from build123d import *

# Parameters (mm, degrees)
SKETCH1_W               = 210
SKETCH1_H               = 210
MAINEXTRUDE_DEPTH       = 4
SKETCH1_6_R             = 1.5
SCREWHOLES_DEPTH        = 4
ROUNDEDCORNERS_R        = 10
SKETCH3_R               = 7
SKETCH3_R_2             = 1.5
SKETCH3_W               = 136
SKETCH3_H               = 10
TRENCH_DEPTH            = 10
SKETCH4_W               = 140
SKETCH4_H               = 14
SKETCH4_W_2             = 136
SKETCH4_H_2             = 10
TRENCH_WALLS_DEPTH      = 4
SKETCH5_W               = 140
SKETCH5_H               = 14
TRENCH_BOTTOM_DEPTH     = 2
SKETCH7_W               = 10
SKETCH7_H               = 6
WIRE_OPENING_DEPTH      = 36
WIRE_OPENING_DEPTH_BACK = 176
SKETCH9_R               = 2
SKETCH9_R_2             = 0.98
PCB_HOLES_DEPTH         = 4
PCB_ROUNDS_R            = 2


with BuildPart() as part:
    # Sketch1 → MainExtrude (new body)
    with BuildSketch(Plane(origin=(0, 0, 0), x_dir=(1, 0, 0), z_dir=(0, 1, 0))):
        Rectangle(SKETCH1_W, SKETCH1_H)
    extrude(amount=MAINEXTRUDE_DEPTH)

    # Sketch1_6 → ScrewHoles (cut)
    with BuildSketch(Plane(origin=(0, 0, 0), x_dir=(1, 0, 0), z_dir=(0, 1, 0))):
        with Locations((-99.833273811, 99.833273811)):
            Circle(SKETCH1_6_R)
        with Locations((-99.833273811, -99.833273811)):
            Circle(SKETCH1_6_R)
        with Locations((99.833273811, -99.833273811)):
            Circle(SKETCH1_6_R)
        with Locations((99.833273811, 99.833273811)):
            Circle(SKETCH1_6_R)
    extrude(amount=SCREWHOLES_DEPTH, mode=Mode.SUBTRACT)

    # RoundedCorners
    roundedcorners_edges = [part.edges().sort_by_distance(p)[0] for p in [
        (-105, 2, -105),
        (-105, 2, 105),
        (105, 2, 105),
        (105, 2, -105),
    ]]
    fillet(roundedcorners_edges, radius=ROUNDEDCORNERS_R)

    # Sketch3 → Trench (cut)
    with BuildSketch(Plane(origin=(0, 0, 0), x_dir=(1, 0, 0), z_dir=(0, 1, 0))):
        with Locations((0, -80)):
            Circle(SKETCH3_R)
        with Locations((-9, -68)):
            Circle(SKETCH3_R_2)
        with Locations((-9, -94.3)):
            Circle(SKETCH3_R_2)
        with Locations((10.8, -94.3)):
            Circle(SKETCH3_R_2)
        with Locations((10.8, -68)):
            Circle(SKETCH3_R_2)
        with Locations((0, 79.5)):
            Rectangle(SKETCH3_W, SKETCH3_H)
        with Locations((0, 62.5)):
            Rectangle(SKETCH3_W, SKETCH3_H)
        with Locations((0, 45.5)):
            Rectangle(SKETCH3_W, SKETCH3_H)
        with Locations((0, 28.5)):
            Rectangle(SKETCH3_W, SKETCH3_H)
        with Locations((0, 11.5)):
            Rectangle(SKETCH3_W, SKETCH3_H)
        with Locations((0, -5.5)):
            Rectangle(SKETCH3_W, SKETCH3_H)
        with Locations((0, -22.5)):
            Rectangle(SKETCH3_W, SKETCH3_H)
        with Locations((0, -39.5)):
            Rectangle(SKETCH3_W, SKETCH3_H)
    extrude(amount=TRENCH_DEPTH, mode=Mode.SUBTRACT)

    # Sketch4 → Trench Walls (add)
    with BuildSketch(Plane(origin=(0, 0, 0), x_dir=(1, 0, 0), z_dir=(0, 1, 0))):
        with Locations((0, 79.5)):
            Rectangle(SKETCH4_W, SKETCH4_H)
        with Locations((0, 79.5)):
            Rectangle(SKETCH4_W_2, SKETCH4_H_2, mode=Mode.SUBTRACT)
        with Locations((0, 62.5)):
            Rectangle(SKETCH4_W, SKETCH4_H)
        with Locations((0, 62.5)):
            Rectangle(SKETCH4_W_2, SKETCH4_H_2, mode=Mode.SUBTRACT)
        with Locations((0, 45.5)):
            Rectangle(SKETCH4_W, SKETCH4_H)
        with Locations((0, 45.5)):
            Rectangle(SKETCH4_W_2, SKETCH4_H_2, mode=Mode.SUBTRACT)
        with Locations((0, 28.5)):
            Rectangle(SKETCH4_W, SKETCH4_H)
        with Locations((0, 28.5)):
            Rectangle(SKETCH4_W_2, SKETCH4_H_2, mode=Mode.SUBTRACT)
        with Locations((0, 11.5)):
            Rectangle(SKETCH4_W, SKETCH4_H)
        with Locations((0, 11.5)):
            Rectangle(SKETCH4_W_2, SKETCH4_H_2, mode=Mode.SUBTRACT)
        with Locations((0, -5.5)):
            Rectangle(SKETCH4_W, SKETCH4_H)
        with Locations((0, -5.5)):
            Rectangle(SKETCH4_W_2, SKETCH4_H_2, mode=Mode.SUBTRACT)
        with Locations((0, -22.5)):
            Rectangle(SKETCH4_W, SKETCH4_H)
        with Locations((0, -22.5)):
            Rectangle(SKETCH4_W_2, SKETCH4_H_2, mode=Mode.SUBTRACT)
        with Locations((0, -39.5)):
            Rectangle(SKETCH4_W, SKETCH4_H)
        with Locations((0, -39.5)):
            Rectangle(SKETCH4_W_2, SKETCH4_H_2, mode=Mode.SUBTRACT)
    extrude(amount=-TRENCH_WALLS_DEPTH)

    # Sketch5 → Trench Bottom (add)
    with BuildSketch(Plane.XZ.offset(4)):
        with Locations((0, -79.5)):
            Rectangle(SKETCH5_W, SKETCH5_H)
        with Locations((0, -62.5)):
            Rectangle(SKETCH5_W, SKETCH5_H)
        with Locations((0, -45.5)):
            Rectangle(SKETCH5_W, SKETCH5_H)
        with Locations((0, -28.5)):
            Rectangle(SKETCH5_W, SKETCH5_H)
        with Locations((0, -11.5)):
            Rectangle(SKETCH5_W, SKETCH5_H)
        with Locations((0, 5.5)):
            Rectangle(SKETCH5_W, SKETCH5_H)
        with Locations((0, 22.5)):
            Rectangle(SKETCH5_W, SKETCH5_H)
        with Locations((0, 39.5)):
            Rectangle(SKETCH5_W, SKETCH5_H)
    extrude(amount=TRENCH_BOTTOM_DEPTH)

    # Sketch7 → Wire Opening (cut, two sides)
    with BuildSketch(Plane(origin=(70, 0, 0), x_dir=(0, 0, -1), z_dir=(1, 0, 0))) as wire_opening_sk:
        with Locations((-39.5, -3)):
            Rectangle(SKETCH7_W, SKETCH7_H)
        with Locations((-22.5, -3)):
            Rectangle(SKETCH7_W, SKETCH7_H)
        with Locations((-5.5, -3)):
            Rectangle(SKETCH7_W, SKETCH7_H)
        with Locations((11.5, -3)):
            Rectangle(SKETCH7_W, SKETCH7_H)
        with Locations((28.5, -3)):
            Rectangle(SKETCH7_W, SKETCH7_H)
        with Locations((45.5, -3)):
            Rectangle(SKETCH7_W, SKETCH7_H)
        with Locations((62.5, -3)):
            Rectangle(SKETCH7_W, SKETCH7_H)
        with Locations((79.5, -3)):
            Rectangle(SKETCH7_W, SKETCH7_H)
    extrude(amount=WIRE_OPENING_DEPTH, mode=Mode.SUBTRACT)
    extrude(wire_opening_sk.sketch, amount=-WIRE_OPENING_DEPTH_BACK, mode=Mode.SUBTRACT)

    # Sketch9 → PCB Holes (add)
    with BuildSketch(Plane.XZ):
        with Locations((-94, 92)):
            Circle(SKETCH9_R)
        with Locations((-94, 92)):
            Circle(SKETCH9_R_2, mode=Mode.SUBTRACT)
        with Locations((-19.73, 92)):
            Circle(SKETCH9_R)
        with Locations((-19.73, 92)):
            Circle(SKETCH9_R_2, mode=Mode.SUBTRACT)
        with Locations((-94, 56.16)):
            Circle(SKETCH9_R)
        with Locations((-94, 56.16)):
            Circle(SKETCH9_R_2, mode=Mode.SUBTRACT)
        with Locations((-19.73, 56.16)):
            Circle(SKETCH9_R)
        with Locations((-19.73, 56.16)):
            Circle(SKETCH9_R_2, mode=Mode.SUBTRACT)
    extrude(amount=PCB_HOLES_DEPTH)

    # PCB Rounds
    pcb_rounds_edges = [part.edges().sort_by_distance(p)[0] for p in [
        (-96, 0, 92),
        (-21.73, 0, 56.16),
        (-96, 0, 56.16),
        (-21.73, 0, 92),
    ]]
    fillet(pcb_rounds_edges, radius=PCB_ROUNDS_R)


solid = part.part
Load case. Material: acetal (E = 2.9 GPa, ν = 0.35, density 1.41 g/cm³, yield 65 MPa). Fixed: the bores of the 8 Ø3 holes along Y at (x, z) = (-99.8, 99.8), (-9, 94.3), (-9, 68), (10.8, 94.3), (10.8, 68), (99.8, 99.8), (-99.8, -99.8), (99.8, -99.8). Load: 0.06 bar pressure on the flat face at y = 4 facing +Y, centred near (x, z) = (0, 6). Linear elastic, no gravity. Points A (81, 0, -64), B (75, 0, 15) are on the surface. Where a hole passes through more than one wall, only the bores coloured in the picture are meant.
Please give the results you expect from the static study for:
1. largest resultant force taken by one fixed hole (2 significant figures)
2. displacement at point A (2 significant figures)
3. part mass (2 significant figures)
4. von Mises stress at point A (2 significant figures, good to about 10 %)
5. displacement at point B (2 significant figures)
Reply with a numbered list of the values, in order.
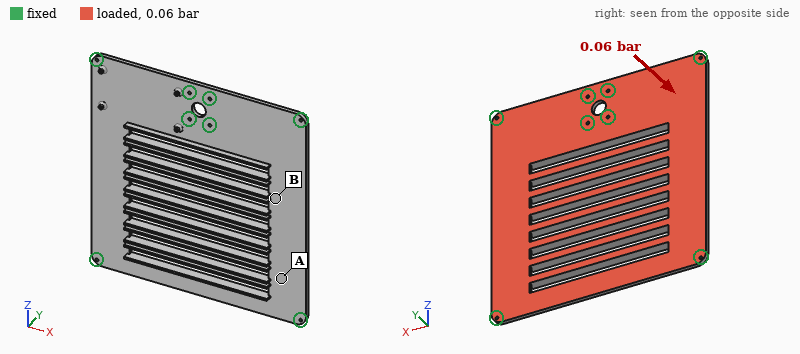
1. 50 N
2. 1.3 mm
3. 220 g
4. 1.7 MPa
5. 2.1 mm
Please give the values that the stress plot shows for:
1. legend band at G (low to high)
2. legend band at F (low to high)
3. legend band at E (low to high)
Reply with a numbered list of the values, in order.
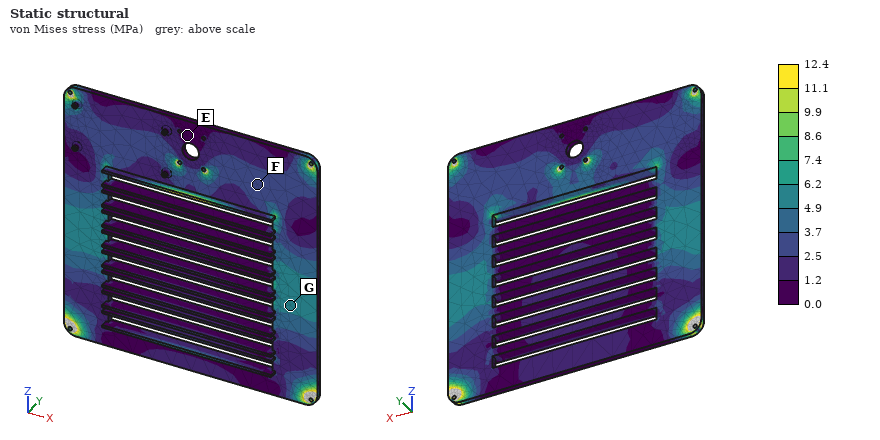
1. 4.9 to 6.2 MPa
2. 2.5 to 3.7 MPa
3. 0.0 to 1.2 MPa
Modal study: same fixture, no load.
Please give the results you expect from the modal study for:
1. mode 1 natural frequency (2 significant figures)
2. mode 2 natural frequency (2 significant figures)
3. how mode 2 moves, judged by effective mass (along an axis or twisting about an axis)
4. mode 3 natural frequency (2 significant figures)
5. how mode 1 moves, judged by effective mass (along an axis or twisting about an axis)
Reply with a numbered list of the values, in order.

1. 99 Hz
2. 150 Hz
3. twisting about Z
4. 190 Hz
5. along Y
